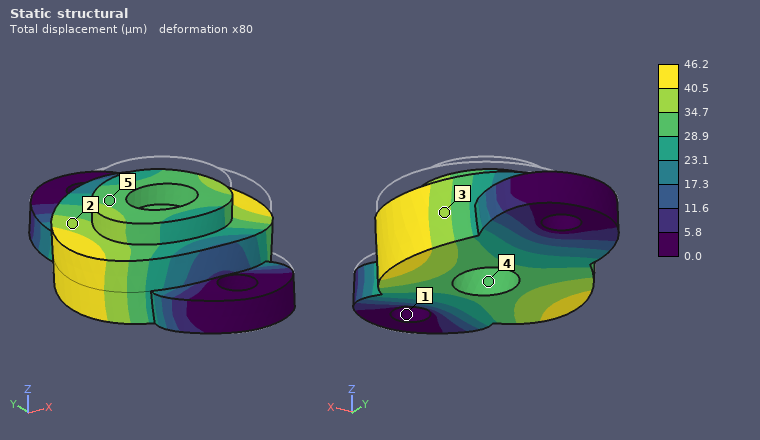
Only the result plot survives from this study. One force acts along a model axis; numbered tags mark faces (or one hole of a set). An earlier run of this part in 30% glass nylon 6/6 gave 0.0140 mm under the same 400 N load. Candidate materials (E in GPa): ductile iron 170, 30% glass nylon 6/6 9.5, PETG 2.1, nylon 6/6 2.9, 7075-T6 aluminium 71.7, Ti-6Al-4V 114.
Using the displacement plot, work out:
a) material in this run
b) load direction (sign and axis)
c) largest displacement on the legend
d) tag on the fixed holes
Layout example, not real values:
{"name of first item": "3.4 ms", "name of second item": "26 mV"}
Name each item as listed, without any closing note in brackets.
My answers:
{"material in this run": "nylon 6/6", "load direction": "-Z", "largest displacement on the legend": "46.2 µm", "tag on the fixed holes": "1"}
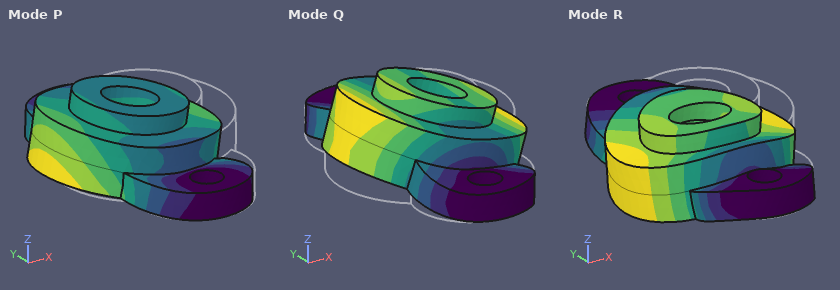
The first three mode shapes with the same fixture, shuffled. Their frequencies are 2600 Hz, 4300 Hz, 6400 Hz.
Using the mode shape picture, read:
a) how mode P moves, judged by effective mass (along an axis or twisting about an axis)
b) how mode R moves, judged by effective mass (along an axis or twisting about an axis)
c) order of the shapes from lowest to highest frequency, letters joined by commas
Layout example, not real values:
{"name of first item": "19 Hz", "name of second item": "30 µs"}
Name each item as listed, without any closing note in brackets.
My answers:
{"how mode P moves, judged by effective mass": "along X", "how mode R moves, judged by effective mass": "along Z", "order of the shapes from lowest to highest frequency, letters joined by commas": "Q, R, P"}
